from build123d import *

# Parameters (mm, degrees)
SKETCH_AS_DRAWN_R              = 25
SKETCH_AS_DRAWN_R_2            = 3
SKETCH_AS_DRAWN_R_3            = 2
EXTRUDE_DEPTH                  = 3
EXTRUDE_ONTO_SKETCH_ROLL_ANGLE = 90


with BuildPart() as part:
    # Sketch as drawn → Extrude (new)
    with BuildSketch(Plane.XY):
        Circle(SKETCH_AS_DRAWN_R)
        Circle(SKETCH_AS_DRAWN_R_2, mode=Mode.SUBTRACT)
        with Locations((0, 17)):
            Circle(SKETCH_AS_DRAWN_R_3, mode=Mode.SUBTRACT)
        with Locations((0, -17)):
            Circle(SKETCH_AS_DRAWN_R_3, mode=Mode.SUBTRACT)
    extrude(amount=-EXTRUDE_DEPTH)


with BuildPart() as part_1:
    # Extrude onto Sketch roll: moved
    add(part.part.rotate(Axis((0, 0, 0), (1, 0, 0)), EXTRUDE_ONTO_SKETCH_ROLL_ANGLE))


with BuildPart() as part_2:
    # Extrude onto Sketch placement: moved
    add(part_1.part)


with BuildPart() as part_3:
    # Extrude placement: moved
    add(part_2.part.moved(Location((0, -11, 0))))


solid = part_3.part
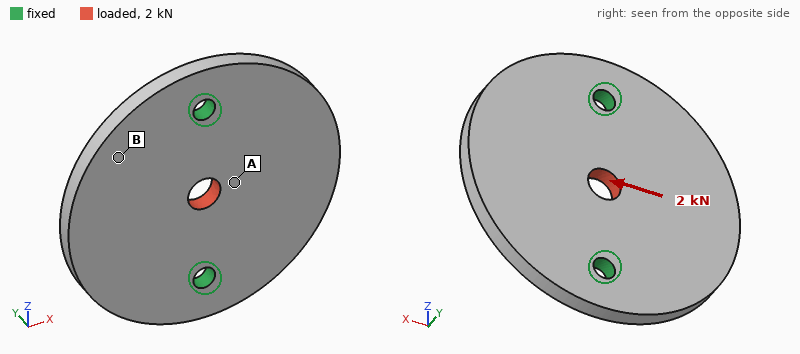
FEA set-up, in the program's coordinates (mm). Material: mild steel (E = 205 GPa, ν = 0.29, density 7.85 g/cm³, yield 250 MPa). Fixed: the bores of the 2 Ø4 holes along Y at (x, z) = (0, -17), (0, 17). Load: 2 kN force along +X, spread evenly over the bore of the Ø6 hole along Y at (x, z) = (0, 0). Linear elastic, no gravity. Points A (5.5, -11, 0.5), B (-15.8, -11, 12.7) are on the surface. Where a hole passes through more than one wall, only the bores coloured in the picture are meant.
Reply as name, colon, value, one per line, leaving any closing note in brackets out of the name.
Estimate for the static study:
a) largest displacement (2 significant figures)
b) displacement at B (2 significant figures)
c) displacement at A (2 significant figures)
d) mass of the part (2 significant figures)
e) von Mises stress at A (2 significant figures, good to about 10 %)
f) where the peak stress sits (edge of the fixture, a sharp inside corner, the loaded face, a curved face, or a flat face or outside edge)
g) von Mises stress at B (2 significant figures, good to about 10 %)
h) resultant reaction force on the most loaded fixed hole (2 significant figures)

largest displacement: 2.9 µm
displacement at B: 1.2 µm
displacement at A: 2.5 µm
mass of the part: 45 g
von Mises stress at A: 30 MPa
where the peak stress sits: edge of the fixture
von Mises stress at B: 9.4 MPa
resultant reaction force on the most loaded fixed hole: 1.0 kN
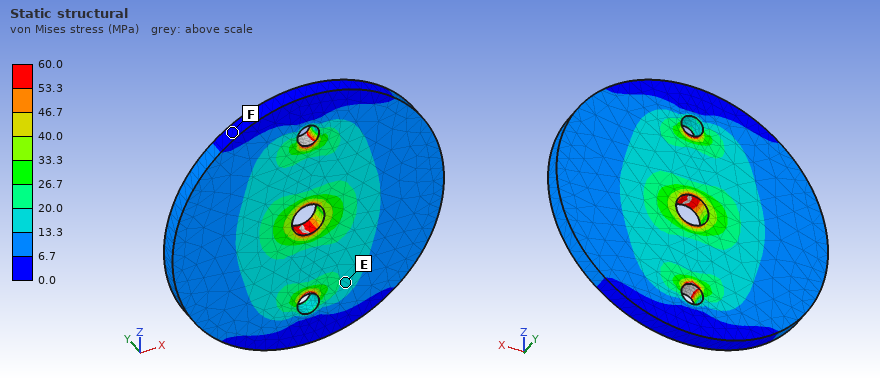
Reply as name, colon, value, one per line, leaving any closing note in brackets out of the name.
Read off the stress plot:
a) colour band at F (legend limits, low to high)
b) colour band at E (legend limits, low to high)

colour band at F: 0.0 to 6.7 MPa
colour band at E: 13.3 to 20.0 MPa
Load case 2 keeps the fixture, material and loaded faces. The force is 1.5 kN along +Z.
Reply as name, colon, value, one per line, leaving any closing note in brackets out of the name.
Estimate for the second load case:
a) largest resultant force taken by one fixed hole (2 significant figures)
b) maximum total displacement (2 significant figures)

largest resultant force taken by one fixed hole: 750 N
maximum total displacement: 1.6 µm
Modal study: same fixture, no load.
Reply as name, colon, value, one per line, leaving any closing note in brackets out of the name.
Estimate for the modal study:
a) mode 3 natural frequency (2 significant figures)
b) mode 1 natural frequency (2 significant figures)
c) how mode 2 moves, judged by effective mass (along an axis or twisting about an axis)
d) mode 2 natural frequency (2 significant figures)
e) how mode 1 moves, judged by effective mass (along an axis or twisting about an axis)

mode 3 natural frequency: 10 kHz
mode 1 natural frequency: 4100 Hz
how mode 2 moves, judged by effective mass: along Y
mode 2 natural frequency: 5000 Hz
how mode 1 moves, judged by effective mass: twisting about Z
